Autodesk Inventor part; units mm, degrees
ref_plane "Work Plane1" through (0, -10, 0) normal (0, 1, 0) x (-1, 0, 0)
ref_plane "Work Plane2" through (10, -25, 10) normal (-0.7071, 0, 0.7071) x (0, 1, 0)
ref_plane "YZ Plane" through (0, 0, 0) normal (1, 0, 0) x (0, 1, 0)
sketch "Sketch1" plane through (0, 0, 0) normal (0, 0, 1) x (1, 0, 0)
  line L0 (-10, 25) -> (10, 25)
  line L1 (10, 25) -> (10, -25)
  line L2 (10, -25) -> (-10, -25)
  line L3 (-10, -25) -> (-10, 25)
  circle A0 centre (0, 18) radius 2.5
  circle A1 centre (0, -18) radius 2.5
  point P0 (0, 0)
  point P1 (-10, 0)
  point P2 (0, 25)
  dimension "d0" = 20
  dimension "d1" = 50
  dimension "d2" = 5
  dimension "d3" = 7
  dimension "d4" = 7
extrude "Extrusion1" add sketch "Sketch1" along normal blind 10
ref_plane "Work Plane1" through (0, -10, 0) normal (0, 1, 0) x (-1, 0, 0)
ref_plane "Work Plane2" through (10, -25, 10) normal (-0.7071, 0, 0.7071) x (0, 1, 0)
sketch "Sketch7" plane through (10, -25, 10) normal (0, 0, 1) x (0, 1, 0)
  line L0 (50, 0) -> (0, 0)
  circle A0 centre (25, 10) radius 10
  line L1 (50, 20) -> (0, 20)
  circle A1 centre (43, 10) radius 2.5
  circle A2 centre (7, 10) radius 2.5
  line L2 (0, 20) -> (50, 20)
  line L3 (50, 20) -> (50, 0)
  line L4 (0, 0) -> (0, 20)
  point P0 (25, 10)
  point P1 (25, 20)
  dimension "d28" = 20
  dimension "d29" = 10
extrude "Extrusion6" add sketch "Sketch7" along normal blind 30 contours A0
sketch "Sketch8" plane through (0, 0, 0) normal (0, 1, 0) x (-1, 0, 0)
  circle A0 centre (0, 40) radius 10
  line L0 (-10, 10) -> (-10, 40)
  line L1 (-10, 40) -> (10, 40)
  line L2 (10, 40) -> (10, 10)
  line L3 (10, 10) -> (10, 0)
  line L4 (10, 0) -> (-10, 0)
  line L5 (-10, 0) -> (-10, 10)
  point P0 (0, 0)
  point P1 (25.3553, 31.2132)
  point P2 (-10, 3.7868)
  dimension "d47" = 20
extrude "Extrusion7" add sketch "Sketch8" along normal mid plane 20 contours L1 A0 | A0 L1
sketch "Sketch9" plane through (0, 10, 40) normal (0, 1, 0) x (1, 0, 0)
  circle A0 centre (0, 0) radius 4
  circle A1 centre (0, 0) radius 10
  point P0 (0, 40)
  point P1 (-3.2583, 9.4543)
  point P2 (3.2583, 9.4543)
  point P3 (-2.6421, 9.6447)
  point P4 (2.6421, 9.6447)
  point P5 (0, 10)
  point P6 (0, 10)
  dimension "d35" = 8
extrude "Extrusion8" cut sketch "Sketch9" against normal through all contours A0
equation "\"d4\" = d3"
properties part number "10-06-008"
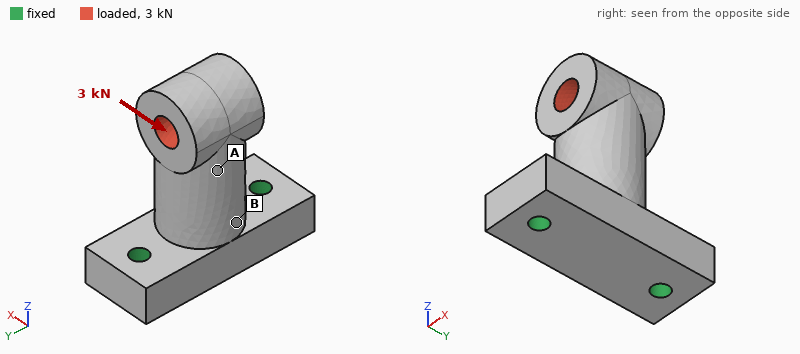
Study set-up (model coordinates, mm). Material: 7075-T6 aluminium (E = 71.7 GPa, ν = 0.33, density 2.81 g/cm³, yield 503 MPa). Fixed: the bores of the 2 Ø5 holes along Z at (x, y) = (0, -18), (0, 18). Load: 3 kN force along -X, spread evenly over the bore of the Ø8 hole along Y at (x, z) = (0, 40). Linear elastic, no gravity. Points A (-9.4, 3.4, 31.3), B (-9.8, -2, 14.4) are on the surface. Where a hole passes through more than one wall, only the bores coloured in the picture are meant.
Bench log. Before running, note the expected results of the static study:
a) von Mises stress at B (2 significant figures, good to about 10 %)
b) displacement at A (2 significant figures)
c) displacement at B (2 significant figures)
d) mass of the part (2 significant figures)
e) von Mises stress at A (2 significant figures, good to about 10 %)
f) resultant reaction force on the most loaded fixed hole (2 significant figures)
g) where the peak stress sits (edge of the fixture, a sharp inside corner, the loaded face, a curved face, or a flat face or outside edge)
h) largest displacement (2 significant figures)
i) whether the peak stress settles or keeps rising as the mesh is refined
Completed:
88 MPa
0.19 mm
0.082 mm
61 g
37 MPa
1.5 kN
edge of the fixture
0.33 mm
keeps rising
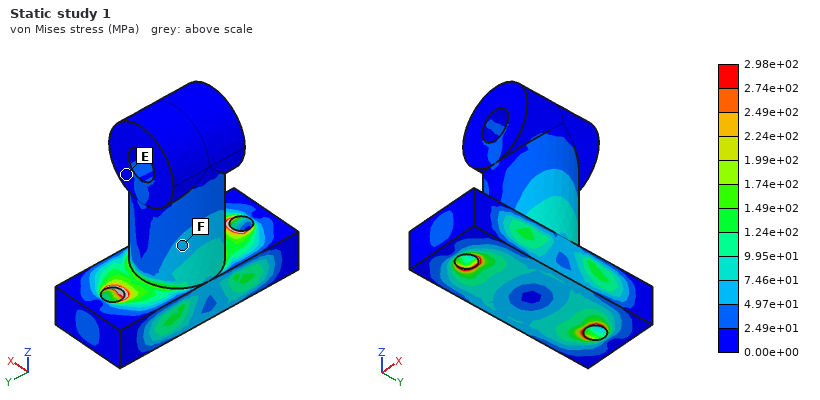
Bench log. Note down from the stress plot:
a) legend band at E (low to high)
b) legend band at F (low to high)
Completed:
0.00e+00 to 2.49e+01 MPa
4.97e+01 to 7.46e+01 MPa
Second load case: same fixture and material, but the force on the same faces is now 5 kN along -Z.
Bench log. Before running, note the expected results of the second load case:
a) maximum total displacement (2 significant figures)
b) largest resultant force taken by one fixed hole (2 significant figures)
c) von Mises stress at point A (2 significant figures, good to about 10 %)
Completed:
20 µm
2.6 kN
18 MPa
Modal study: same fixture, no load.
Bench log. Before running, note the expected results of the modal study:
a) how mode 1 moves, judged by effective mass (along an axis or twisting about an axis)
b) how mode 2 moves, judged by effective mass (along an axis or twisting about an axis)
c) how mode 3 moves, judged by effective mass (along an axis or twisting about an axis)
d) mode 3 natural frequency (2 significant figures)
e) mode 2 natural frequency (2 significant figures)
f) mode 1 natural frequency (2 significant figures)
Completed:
along X
along Y
along Z
15 kHz
6200 Hz
3900 Hz
